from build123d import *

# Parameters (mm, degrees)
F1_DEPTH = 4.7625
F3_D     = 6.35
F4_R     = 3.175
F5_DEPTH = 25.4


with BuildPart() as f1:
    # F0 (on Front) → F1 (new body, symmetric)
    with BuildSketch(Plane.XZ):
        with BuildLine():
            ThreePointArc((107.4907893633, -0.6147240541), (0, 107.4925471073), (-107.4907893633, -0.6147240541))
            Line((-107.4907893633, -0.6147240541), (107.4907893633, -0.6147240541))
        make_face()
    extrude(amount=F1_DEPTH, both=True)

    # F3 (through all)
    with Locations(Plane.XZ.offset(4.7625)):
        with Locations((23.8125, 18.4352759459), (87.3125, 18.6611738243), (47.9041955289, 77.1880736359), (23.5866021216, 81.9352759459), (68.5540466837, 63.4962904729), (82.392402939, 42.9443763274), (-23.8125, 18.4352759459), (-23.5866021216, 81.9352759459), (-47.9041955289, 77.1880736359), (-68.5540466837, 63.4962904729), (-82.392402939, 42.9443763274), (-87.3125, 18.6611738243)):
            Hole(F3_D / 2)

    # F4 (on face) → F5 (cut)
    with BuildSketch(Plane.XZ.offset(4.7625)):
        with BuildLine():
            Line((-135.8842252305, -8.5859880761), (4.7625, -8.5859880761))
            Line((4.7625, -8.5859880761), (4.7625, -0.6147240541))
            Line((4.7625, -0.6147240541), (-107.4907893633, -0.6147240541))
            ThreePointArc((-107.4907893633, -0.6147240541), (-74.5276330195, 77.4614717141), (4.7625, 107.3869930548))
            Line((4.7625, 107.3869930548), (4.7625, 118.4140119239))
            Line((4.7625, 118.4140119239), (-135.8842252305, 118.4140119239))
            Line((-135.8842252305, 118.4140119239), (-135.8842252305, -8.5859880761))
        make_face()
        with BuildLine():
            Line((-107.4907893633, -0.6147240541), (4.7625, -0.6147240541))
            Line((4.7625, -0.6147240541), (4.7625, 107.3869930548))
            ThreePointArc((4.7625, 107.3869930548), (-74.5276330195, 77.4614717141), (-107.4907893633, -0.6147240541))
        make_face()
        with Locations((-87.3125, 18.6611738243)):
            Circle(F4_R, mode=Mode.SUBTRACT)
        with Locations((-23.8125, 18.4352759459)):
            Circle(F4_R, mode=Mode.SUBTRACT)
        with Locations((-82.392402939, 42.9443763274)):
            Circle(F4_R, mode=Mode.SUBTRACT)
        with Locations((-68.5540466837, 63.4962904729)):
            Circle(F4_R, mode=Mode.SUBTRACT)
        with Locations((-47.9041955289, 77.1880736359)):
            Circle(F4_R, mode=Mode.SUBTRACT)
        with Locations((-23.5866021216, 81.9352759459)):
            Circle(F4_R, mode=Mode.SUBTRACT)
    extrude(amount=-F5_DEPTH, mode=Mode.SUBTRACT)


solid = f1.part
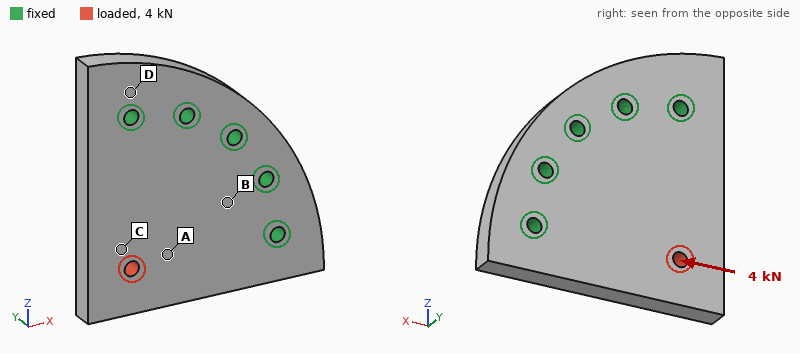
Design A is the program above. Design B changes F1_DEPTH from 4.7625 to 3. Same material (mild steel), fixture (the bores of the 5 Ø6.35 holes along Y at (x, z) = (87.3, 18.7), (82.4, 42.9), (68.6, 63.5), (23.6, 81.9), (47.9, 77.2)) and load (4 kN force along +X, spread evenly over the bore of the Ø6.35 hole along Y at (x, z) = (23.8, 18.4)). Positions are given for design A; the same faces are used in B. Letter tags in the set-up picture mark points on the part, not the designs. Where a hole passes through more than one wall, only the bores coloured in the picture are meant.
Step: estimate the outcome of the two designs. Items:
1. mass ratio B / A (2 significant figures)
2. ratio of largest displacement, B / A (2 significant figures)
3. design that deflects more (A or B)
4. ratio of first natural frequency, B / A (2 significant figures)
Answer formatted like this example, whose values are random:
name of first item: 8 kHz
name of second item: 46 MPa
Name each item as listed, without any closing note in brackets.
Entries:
mass ratio B / A: 0.63
ratio of largest displacement, B / A: 1.6
design that deflects more: B
ratio of first natural frequency, B / A: 0.65
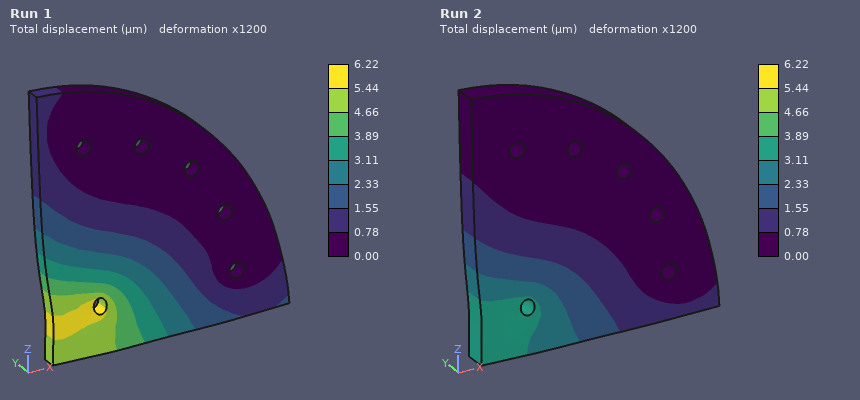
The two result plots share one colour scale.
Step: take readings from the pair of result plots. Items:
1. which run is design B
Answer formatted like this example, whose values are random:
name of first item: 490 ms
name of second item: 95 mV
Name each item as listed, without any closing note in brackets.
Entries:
which run is design B: Run 1
